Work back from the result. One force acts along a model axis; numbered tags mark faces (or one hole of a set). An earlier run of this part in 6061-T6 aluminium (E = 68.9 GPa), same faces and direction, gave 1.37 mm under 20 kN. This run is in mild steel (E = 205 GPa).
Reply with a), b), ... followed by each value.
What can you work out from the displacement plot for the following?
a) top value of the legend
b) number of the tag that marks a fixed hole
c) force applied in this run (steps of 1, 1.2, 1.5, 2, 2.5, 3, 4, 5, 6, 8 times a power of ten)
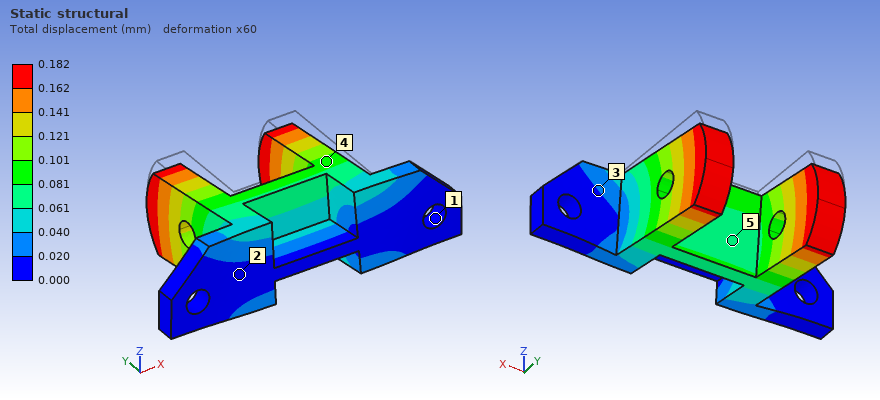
a) 0.182 mm
b) 1
c) 8 kN
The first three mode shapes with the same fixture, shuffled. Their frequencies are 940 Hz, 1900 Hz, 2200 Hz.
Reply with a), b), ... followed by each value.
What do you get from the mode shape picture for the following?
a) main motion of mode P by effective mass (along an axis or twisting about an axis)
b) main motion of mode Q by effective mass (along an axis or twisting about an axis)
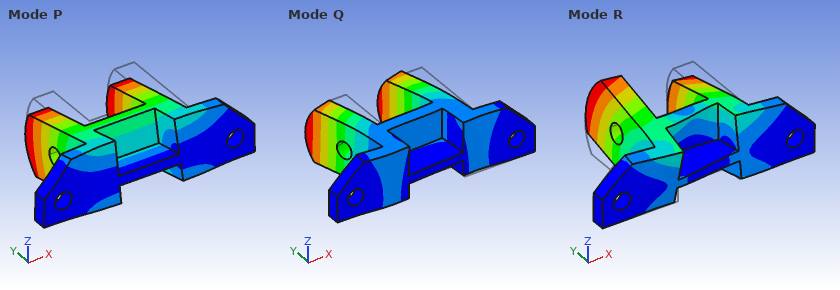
a) along Z
b) along X
